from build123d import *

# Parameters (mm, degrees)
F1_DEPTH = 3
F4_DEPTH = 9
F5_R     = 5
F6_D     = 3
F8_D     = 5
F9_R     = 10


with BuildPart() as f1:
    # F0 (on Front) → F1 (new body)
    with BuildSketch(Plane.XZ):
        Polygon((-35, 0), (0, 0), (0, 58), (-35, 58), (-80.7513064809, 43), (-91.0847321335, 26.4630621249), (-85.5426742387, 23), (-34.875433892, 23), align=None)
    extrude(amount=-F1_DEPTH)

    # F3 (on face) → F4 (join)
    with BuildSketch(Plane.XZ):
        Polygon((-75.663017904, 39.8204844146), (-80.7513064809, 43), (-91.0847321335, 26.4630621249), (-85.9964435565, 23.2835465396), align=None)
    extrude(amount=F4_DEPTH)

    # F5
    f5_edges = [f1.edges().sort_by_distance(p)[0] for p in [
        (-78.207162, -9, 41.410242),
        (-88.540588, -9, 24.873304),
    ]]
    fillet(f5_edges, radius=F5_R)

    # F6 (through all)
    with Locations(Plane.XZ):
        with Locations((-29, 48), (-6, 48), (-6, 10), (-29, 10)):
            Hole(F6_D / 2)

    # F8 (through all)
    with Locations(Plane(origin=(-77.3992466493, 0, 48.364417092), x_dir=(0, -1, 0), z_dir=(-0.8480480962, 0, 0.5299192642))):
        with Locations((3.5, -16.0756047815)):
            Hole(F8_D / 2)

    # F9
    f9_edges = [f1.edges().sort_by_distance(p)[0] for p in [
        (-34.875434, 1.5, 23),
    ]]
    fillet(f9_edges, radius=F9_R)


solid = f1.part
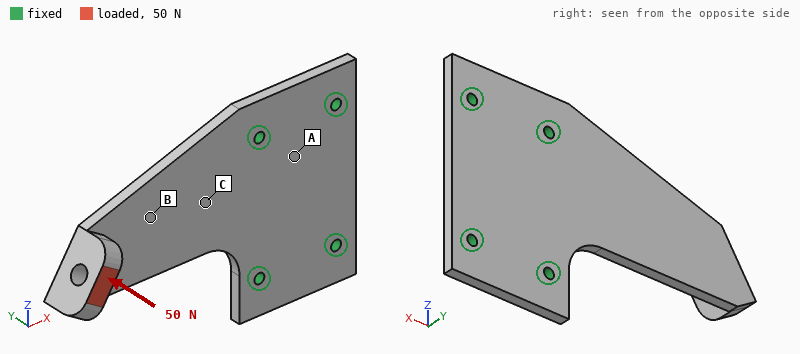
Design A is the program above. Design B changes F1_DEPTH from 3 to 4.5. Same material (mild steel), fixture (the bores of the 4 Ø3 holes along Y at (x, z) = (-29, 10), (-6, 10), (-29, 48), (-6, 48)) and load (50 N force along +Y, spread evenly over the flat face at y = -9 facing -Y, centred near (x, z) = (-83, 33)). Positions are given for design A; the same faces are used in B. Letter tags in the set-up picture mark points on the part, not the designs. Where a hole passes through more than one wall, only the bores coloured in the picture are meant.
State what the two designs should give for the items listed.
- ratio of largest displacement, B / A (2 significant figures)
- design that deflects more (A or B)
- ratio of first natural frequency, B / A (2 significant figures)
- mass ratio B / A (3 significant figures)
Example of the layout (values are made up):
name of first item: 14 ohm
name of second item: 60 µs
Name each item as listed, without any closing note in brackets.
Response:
ratio of largest displacement, B / A: 0.30
design that deflects more: A
ratio of first natural frequency, B / A: 1.6
mass ratio B / A: 1.46
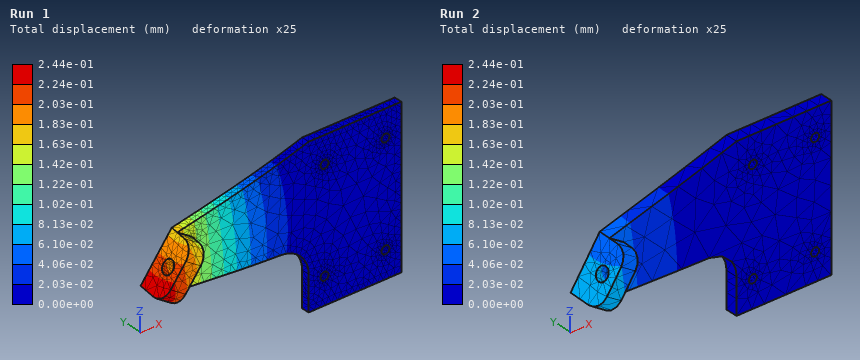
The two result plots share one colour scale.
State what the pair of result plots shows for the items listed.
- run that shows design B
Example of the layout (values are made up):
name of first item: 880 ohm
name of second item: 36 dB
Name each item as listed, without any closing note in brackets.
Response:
run that shows design B: Run 2
